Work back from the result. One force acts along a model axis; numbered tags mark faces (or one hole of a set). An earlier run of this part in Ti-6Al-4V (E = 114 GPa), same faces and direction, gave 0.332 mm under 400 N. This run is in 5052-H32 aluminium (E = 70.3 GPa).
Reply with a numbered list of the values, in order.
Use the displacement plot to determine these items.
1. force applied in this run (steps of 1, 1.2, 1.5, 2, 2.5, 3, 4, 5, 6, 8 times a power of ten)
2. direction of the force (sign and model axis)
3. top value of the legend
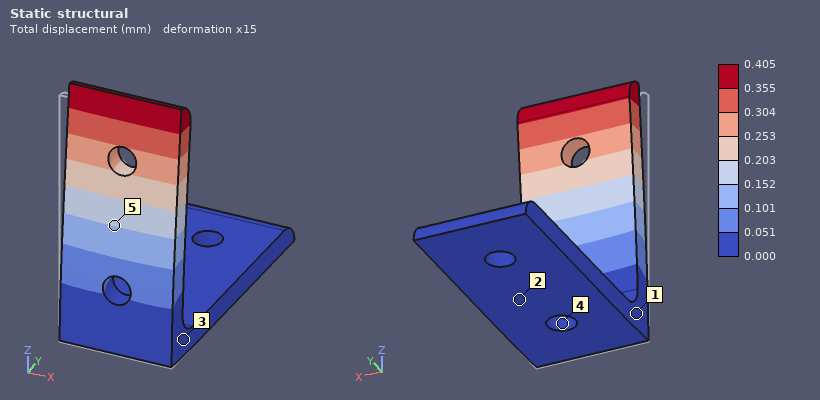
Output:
1. 300 N
2. +Y
3. 0.405 mm
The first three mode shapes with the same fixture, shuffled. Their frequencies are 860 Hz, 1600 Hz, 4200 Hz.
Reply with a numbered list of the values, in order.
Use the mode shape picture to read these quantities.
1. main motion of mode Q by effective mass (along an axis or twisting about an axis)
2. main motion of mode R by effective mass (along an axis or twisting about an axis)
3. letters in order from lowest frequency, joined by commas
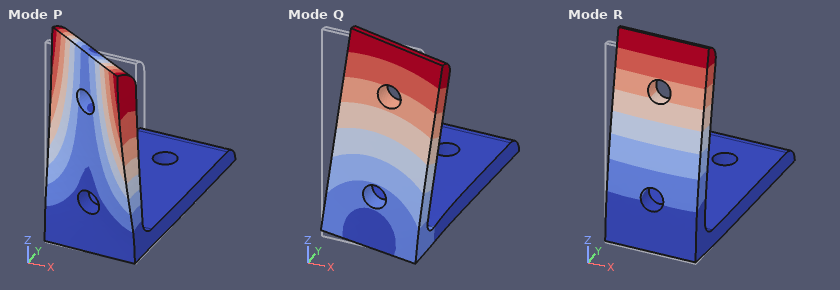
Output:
1. along X
2. along Y
3. R, Q, P
